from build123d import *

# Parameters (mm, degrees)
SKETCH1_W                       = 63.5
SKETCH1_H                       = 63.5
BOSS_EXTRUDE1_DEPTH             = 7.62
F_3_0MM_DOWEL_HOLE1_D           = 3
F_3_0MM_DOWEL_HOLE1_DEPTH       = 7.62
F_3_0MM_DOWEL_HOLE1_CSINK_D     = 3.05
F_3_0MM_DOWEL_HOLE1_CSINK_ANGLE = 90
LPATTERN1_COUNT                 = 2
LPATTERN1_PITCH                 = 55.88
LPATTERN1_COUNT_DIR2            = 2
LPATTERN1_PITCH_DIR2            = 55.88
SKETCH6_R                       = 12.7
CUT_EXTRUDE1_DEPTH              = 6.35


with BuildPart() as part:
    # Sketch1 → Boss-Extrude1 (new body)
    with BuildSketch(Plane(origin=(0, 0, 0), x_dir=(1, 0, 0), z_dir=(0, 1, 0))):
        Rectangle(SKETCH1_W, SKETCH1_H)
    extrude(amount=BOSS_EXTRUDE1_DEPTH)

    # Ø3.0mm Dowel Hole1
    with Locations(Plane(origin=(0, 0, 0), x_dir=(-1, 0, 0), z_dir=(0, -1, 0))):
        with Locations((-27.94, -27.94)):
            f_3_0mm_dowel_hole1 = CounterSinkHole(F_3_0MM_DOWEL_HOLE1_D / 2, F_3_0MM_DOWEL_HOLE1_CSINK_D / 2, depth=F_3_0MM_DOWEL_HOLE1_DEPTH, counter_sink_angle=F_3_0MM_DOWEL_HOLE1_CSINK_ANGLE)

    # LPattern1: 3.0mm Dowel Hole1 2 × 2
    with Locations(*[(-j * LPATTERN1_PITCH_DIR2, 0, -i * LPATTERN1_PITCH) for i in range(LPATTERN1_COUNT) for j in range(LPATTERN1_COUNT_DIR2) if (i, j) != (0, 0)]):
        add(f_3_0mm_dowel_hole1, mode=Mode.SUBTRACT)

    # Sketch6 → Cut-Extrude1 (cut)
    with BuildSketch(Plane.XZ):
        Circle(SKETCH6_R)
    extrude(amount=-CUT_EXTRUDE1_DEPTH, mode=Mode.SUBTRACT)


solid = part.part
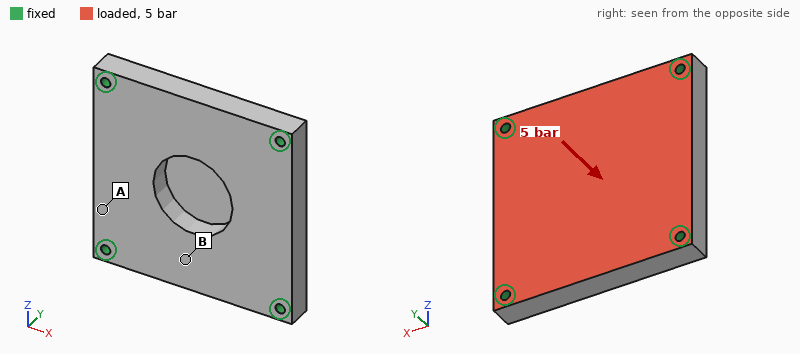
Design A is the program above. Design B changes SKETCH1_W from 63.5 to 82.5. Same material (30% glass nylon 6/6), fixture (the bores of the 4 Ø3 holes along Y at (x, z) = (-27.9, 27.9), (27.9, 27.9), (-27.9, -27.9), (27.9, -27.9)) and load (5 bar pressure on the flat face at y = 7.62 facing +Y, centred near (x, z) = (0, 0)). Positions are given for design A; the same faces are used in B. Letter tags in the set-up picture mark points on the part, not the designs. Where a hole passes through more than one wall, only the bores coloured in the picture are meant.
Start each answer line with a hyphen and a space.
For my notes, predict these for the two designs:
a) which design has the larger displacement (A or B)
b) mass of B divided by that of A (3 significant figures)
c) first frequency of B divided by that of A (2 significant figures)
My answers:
- A
- 1.34
- 1.0
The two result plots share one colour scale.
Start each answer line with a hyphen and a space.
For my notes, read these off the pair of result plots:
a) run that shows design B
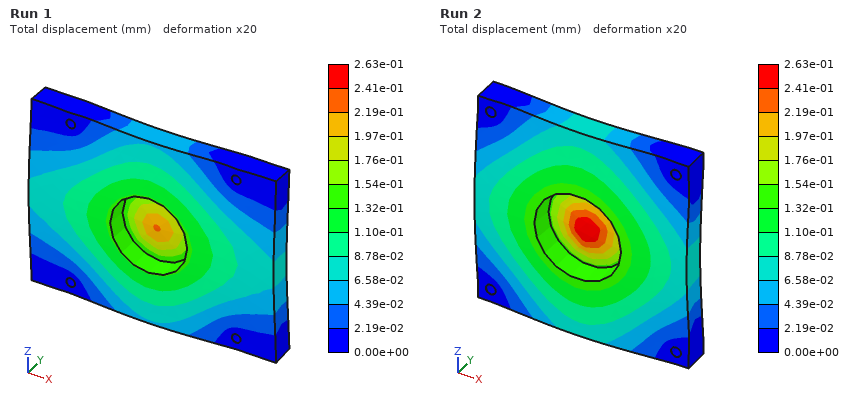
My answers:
- Run 1
